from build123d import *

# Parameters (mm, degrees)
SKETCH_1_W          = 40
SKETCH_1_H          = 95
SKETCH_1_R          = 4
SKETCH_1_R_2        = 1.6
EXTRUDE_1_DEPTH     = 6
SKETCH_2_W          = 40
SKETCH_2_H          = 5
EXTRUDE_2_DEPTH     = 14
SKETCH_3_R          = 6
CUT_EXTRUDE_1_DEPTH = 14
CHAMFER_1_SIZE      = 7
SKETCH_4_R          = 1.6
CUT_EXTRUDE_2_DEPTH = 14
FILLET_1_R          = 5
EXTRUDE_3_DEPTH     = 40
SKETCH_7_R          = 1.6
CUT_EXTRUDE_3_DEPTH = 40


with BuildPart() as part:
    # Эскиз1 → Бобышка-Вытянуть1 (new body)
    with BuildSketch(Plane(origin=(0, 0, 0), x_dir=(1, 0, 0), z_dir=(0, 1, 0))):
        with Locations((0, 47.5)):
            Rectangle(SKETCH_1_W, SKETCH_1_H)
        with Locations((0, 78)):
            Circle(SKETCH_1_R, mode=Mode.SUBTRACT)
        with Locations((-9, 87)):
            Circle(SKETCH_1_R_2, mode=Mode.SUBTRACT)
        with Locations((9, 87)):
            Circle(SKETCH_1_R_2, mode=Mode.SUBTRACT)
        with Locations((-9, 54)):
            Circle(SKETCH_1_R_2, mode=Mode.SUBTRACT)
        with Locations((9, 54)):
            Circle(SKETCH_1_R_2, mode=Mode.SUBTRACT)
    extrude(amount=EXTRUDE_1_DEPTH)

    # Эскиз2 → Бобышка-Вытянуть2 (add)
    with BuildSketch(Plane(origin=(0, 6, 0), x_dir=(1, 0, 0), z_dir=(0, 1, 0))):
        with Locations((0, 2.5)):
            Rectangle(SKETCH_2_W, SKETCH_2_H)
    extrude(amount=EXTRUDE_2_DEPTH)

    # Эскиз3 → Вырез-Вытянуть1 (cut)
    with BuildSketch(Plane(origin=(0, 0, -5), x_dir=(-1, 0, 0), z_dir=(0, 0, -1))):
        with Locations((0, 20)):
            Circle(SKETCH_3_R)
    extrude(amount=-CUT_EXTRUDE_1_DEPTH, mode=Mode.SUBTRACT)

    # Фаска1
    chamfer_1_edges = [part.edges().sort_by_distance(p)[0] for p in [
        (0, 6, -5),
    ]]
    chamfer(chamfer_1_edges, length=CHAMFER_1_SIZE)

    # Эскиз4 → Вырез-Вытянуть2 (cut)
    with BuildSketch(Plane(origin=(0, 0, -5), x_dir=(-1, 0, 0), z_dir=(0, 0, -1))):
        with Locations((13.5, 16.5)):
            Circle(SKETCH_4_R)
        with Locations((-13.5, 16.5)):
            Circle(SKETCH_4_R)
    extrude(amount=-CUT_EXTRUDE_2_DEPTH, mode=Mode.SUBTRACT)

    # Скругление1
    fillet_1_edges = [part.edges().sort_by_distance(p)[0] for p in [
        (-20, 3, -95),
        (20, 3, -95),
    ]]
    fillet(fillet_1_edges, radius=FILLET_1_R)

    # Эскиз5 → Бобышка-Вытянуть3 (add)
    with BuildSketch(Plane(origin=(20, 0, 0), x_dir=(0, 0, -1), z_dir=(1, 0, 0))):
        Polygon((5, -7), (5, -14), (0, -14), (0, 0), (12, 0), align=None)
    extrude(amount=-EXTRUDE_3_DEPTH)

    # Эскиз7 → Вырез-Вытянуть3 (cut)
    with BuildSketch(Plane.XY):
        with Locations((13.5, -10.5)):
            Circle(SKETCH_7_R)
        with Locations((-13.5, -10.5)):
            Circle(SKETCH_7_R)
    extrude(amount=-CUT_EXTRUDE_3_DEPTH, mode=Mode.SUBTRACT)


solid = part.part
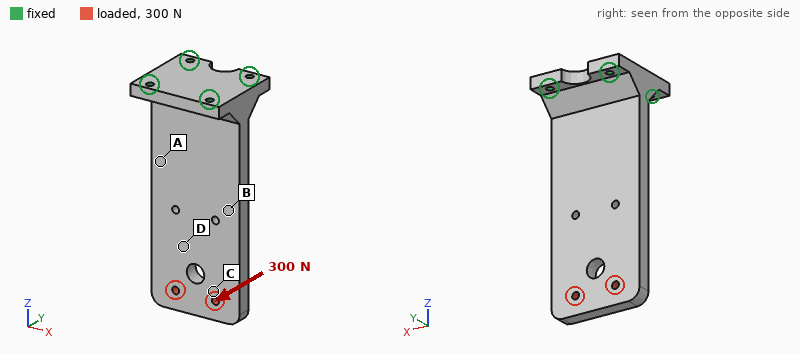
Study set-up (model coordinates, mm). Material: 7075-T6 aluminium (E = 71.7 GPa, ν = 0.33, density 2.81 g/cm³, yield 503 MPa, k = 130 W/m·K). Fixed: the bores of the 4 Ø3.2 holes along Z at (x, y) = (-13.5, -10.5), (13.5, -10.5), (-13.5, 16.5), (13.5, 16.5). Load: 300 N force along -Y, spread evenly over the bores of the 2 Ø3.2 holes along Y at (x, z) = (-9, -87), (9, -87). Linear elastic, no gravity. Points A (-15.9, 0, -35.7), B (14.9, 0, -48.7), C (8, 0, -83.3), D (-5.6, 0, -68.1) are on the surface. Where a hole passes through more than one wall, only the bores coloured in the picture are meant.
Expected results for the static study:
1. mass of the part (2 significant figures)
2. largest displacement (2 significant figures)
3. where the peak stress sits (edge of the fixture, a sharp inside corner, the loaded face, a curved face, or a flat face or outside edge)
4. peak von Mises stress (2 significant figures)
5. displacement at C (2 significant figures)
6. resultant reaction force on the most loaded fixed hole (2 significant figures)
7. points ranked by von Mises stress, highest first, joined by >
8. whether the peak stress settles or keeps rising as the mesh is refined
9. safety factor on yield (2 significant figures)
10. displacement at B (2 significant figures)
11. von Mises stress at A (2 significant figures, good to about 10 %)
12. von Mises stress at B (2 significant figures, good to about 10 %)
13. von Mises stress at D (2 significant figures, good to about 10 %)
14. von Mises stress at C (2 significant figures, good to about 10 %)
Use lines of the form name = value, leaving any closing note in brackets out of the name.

mass of the part = 82 g
largest displacement = 1.0 mm
where the peak stress sits = a curved face
peak von Mises stress = 90 MPa
displacement at C = 0.84 mm
resultant reaction force on the most loaded fixed hole = 560 N
points ranked by von Mises stress, highest first, joined by > = A > B > D > C
whether the peak stress settles or keeps rising as the mesh is refined = settles
safety factor on yield = 5.6
displacement at B = 0.29 mm
von Mises stress at A = 64 MPa
von Mises stress at B = 50 MPa
von Mises stress at D = 25 MPa
von Mises stress at C = 9.5 MPa
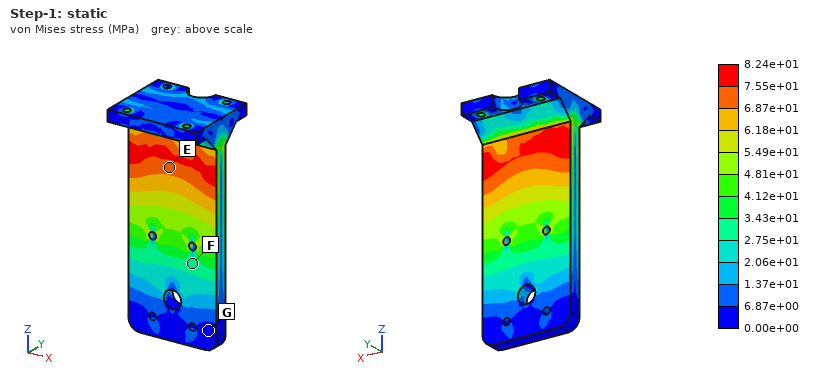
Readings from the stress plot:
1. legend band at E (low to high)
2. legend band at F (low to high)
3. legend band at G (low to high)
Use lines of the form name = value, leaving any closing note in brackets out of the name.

legend band at E = 6.87e+01 to 7.55e+01 MPa
legend band at F = 2.75e+01 to 3.43e+01 MPa
legend band at G = 0.00e+00 to 6.87e+00 MPa
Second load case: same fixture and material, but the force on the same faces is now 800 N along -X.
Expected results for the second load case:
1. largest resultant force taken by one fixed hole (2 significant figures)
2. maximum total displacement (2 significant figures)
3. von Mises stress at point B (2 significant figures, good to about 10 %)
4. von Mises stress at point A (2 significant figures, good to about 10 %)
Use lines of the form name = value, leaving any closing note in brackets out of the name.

largest resultant force taken by one fixed hole = 1.3 kN
maximum total displacement = 0.15 mm
von Mises stress at point B = 15 MPa
von Mises stress at point A = 21 MPa
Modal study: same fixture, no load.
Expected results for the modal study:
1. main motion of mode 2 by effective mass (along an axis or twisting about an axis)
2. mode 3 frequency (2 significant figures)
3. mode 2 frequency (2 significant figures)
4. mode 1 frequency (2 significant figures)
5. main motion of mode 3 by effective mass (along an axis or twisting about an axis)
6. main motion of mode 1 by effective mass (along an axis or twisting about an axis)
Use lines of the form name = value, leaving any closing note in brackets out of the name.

main motion of mode 2 by effective mass = along X
mode 3 frequency = 2900 Hz
mode 2 frequency = 2700 Hz
mode 1 frequency = 690 Hz
main motion of mode 3 by effective mass = twisting about Z
main motion of mode 1 by effective mass = along Y
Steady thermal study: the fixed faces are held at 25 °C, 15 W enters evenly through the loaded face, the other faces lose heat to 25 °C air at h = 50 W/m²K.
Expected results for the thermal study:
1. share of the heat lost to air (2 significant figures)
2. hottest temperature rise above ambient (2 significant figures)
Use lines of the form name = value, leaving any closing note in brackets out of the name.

share of the heat lost to air = 45 %
hottest temperature rise above ambient = 31 K
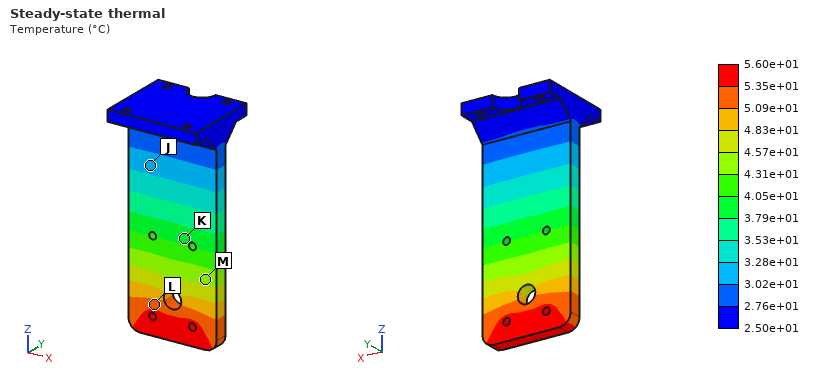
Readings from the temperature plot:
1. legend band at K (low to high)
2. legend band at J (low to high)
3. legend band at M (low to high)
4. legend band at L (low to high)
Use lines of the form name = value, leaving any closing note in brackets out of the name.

legend band at K = 3.79e+01 to 4.05e+01 °C
legend band at J = 3.02e+01 to 3.28e+01 °C
legend band at M = 4.31e+01 to 4.57e+01 °C
legend band at L = 5.09e+01 to 5.35e+01 °C
